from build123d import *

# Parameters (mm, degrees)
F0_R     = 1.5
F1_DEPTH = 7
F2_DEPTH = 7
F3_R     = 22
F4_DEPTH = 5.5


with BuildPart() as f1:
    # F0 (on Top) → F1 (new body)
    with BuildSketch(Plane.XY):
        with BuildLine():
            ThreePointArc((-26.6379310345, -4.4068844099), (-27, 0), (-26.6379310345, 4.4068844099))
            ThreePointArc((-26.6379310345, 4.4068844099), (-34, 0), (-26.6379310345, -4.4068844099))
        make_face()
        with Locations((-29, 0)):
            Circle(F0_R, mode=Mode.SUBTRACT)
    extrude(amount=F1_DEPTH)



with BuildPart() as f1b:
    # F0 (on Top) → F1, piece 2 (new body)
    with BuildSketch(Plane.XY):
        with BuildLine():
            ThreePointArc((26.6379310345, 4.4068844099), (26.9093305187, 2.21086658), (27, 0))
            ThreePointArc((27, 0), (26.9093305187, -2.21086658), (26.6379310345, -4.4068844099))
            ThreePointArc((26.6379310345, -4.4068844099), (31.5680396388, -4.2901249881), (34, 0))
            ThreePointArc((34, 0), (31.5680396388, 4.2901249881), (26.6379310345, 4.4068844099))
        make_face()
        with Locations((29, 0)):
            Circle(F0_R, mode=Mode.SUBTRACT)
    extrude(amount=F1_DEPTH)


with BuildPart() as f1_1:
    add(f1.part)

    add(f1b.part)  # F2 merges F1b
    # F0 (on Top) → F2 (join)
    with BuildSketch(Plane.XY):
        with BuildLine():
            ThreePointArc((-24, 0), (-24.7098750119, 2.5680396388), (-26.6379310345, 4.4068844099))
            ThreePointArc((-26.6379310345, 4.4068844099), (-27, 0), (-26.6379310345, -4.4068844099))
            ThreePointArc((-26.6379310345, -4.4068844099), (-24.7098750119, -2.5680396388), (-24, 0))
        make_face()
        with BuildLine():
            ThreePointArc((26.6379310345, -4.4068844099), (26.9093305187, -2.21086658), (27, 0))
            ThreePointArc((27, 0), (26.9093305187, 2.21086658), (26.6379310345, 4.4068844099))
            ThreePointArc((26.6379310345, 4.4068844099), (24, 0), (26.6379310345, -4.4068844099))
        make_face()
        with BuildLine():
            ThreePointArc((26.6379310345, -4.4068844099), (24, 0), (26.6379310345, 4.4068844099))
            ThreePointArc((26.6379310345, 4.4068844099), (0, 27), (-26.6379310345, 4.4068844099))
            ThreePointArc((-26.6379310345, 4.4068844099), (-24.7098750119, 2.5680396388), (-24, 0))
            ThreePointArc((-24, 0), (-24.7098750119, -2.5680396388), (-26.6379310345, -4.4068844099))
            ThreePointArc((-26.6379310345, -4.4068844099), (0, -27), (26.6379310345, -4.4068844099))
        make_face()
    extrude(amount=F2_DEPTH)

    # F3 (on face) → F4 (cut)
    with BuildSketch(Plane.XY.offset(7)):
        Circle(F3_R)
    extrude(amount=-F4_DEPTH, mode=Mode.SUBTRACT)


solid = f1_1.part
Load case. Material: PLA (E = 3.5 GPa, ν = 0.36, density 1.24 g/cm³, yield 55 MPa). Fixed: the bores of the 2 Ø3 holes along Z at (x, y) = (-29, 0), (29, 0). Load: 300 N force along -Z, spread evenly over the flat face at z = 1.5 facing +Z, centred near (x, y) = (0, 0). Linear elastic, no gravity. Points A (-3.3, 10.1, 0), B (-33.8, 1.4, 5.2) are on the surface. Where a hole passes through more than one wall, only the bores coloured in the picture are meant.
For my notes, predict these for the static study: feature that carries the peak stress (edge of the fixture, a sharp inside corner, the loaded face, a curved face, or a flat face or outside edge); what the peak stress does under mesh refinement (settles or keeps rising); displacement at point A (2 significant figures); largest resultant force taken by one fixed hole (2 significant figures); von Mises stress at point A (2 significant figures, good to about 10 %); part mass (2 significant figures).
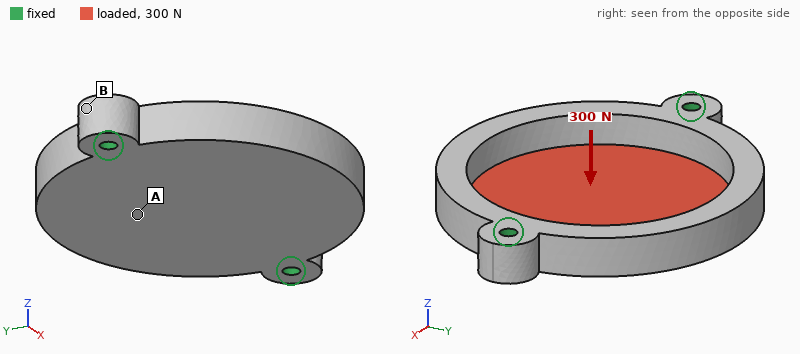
edge of the fixture
keeps rising
0.69 mm
180 N
17 MPa
10 g
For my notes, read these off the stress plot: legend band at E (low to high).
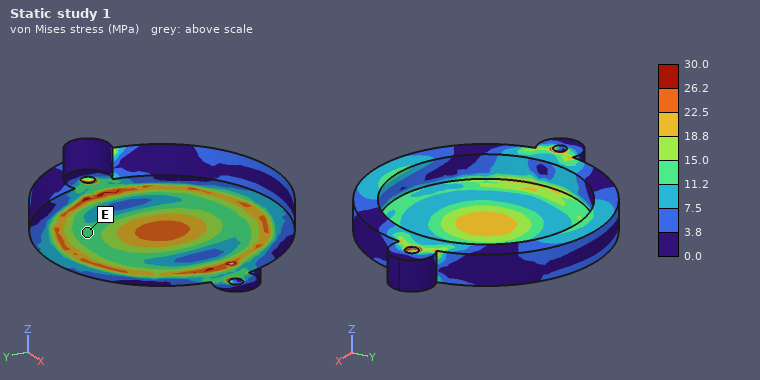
11.2 to 15.0 MPa
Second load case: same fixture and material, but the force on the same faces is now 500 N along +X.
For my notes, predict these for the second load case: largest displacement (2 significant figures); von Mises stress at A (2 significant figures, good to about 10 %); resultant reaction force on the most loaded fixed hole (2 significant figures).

45 µm
1.7 MPa
250 N
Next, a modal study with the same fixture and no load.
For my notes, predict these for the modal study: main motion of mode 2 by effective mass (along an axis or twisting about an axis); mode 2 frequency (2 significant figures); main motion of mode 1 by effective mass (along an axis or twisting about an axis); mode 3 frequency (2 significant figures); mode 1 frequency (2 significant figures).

along Z
1700 Hz
twisting about X
2500 Hz
1400 Hz
